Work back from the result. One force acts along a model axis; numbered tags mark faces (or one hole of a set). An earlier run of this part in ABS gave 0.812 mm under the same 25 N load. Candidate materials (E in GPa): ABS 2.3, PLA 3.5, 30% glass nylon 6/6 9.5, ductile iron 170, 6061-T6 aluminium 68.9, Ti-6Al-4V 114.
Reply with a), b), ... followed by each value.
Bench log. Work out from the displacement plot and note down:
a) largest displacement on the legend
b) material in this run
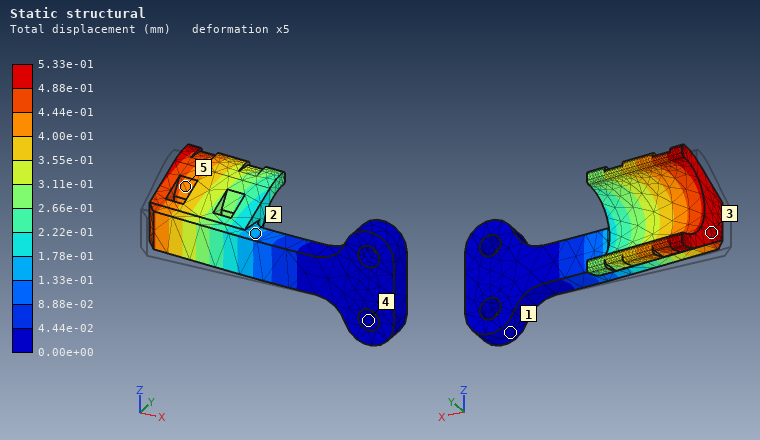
a) 5.33e-01 mm
b) PLA
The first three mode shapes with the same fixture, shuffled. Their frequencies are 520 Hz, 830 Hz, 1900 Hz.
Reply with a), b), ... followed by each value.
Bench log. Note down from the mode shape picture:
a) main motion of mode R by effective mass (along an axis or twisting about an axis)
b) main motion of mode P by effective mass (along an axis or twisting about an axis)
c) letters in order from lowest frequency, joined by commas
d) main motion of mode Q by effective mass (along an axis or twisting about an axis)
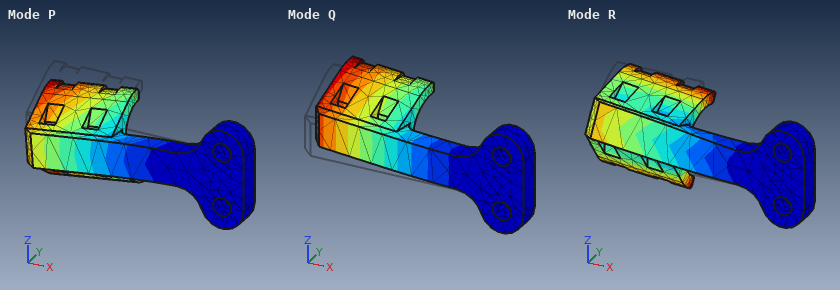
a) twisting about X
b) along Z
c) Q, P, R
d) along Y
